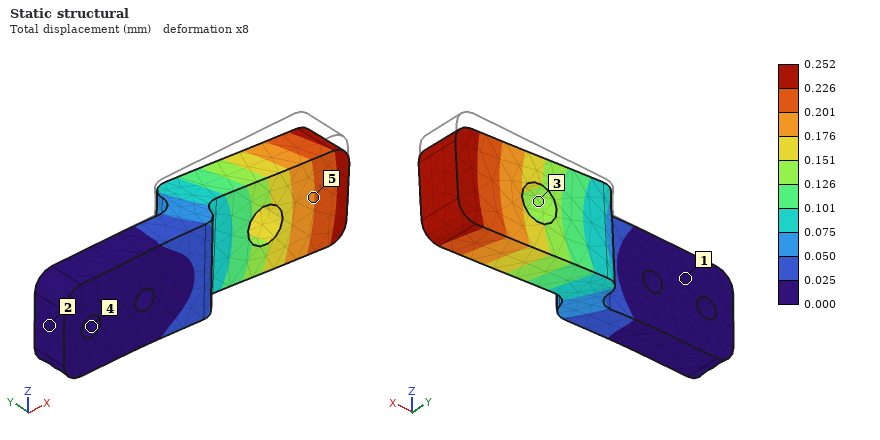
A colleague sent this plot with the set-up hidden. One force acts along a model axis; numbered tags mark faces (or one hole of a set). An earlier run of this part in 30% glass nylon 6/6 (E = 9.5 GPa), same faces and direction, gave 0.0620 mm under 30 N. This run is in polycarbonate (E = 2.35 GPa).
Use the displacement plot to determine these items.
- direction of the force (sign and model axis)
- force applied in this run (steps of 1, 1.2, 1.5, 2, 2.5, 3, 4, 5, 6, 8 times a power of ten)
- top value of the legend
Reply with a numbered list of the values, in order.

1. -Z
2. 30 N
3. 0.252 mm
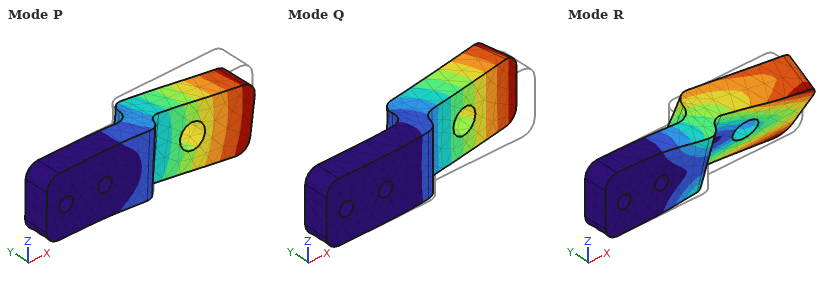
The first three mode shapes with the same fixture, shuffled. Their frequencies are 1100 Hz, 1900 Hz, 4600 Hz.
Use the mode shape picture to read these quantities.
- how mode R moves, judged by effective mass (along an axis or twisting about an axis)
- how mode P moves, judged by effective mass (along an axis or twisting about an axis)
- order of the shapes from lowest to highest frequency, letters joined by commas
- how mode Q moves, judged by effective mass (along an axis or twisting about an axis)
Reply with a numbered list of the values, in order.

1. twisting about X
2. along Z
3. Q, P, R
4. along Y
